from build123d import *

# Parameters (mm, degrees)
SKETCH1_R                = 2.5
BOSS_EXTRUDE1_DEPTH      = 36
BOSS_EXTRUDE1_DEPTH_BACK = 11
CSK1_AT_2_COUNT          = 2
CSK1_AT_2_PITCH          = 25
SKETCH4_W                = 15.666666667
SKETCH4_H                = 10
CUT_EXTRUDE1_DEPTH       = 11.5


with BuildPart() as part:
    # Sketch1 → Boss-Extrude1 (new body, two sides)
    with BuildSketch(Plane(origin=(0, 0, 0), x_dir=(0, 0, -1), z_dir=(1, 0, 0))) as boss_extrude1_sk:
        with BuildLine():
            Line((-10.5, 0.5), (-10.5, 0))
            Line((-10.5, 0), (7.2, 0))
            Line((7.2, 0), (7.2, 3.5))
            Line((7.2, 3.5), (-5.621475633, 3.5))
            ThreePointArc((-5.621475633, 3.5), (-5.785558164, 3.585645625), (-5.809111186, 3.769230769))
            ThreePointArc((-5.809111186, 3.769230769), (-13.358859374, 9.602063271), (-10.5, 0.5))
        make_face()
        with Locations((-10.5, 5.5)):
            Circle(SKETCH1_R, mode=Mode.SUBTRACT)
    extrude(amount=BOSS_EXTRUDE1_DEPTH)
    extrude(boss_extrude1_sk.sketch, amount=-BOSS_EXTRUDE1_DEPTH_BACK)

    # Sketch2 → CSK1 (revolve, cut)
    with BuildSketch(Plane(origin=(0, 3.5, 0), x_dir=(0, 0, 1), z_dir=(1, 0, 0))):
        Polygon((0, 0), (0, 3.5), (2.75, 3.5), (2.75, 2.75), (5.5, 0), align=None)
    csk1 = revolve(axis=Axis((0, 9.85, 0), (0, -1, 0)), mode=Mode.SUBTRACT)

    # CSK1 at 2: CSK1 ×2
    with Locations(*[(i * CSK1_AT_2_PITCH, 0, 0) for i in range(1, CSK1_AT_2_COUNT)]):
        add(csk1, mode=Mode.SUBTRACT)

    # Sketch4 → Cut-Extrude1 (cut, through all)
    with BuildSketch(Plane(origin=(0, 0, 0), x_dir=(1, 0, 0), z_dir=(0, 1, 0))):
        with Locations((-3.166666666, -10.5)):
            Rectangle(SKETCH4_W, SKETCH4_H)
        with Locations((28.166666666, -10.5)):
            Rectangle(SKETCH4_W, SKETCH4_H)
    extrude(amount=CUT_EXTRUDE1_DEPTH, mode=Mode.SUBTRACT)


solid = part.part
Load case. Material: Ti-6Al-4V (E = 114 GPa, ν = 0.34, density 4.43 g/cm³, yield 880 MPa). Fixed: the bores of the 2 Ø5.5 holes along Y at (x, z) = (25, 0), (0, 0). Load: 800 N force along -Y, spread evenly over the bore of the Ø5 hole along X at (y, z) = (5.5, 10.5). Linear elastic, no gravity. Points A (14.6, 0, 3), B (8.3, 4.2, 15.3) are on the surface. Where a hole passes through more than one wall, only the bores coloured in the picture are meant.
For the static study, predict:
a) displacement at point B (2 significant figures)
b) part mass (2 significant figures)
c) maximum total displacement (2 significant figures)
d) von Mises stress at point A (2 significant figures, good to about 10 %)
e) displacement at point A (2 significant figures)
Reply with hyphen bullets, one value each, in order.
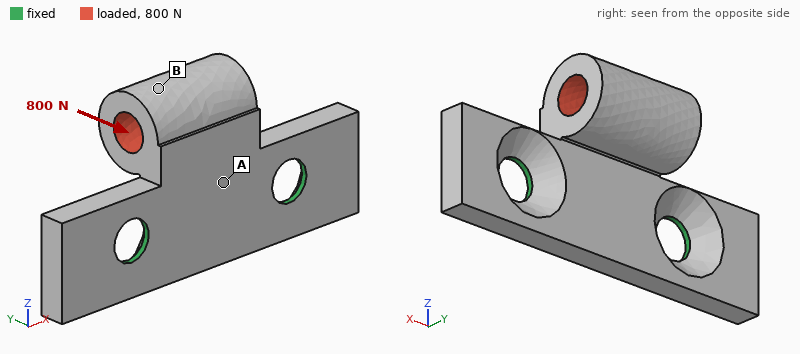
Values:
- 0.17 mm
- 12 g
- 0.18 mm
- 100 MPa
- 0.031 mm
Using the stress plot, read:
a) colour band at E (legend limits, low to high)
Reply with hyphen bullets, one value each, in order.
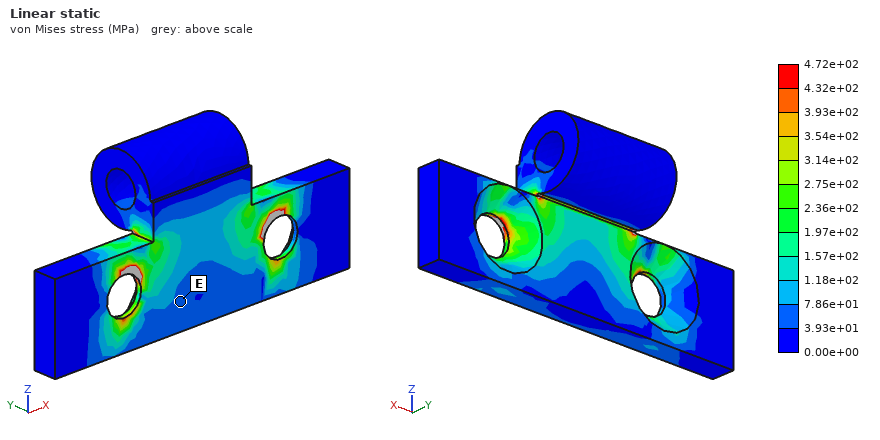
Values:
- 3.93e+01 to 7.86e+01 MPa
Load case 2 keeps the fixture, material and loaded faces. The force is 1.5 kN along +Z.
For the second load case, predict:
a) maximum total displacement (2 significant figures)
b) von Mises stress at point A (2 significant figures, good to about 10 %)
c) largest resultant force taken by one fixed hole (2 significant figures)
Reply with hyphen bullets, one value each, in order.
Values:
- 0.18 mm
- 100 MPa
- 760 N
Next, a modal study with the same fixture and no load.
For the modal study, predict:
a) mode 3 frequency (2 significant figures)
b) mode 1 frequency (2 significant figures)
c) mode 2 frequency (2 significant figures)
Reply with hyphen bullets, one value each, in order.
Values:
- 15 kHz
- 5400 Hz
- 15 kHz
